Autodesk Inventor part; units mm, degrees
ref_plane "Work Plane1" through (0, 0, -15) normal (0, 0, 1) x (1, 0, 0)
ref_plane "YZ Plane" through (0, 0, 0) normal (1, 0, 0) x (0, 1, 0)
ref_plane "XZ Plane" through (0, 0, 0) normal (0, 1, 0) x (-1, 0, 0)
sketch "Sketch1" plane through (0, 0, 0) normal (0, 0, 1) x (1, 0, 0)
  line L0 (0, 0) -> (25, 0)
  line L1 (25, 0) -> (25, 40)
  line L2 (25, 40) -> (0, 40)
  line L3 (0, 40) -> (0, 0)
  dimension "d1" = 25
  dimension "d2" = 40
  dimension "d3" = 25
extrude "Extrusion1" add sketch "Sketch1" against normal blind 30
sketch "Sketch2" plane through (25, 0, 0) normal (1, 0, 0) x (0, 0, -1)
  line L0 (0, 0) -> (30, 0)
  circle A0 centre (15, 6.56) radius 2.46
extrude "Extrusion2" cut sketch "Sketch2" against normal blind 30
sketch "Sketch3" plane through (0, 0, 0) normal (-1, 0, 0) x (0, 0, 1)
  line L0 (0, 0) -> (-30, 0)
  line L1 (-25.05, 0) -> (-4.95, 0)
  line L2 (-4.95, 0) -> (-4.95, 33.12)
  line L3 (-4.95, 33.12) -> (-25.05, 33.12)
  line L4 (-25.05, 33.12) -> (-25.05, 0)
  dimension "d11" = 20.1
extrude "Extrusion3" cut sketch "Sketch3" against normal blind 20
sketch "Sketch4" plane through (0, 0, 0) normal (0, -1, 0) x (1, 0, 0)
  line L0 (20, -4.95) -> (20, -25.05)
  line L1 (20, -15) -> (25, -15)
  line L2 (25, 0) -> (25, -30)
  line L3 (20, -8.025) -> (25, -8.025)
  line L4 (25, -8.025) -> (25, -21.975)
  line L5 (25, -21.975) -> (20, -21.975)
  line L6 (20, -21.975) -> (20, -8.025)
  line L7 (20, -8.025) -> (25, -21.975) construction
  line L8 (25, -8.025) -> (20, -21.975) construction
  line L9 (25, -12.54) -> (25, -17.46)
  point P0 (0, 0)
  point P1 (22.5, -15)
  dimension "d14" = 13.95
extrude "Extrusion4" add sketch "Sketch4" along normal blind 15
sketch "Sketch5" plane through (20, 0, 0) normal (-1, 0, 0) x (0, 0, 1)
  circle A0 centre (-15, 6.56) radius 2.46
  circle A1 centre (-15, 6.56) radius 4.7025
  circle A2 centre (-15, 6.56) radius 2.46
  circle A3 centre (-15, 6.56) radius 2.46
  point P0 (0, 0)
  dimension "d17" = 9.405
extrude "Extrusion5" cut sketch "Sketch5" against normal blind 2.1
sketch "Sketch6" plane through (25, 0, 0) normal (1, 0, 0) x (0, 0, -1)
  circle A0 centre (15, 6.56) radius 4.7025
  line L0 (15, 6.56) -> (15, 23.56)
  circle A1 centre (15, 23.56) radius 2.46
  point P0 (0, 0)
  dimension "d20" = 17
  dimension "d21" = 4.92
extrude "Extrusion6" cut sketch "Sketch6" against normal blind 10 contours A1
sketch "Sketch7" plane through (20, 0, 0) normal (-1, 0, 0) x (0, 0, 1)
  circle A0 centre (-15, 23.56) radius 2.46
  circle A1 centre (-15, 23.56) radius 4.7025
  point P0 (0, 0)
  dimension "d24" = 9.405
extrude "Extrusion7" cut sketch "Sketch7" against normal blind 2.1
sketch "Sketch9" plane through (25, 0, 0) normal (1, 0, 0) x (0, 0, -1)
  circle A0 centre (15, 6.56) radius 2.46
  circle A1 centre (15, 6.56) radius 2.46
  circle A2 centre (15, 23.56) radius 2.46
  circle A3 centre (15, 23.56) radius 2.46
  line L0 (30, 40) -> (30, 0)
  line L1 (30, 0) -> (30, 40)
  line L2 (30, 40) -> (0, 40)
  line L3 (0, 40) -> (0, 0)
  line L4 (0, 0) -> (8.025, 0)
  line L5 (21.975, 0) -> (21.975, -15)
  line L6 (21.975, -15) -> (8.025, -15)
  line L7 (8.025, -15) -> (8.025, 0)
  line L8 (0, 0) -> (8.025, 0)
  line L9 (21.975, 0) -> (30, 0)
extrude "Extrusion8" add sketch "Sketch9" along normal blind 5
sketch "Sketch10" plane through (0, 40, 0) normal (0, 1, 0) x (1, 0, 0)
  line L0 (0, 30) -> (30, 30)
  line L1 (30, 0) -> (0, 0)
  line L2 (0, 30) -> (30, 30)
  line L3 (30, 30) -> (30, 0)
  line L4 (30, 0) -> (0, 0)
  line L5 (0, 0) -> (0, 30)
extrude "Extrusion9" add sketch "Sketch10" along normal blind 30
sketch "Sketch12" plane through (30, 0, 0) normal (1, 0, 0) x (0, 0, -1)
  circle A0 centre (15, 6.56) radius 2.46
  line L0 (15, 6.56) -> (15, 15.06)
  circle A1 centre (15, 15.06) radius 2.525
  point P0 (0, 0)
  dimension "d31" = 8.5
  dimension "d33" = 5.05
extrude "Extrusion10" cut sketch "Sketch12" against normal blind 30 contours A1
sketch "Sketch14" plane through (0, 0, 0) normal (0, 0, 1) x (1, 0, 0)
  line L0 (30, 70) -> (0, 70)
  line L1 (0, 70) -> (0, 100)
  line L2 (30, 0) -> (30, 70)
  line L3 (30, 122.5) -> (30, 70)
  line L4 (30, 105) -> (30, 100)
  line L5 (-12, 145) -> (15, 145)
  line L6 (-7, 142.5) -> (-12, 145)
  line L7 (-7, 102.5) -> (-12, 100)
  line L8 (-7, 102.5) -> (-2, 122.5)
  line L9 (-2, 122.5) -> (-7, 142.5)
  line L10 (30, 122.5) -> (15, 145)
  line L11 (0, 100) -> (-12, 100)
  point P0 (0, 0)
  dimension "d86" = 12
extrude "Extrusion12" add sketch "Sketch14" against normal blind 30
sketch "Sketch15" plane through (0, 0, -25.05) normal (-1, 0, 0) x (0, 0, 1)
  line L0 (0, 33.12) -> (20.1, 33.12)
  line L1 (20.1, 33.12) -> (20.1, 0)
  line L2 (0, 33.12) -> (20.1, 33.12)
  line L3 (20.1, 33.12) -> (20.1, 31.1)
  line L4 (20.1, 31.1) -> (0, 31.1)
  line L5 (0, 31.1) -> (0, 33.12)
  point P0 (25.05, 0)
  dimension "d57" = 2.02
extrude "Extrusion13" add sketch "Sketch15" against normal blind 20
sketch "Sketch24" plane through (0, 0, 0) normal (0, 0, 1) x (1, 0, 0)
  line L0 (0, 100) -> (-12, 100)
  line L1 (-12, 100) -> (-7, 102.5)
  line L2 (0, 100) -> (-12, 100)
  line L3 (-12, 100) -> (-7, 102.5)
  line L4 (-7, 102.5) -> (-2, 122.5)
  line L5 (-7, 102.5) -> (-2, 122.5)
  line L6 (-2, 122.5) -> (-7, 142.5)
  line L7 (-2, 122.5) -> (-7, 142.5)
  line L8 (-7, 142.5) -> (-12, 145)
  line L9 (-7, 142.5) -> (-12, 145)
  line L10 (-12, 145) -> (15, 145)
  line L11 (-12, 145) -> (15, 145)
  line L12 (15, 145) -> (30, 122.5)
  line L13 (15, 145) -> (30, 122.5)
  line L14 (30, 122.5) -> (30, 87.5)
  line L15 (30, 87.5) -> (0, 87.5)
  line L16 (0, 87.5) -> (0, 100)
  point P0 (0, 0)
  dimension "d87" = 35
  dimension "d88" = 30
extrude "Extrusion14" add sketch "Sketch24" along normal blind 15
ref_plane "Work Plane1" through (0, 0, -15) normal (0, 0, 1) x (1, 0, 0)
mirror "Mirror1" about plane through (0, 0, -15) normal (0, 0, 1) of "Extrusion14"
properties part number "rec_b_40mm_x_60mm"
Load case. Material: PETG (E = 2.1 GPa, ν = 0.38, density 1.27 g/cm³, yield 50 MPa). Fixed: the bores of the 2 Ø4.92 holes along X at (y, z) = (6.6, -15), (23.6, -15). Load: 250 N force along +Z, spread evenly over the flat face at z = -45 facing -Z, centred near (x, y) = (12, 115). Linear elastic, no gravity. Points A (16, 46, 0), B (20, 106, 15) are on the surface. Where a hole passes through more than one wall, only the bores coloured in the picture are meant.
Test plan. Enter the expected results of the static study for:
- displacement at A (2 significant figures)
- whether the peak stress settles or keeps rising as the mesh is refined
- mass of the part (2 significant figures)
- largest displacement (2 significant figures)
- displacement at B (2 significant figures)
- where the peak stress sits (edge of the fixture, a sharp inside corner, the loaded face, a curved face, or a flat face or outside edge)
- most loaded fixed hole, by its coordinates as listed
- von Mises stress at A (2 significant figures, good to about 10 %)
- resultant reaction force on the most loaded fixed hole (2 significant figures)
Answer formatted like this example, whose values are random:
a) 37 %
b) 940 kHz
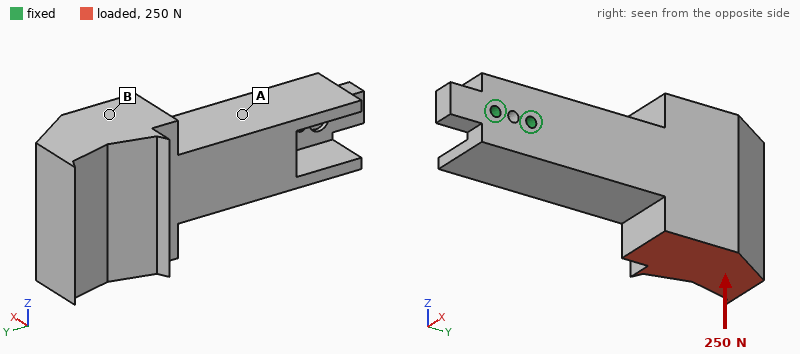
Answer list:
a) 0.35 mm
b) keeps rising
c) 220 g
d) 2.1 mm
e) 1.4 mm
f) edge of the fixture
g) (23.6, -15)
h) 4.2 MPa
i) 1.2 kN
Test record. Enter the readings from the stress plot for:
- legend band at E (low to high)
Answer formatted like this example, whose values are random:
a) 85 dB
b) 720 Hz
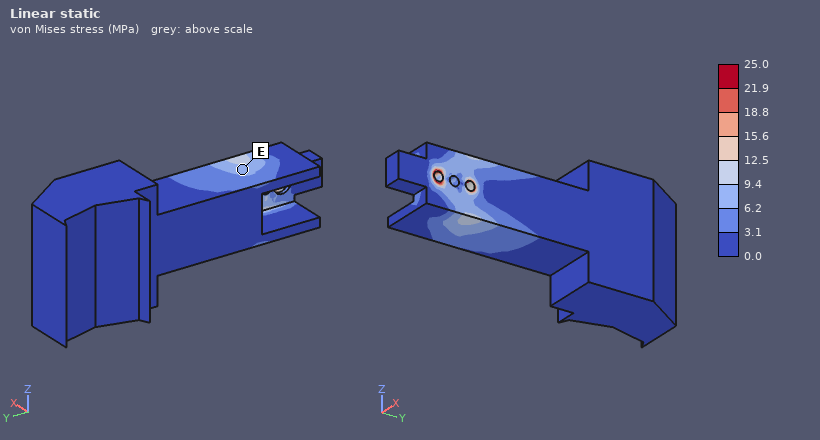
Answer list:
a) 6.2 to 9.4 MPa
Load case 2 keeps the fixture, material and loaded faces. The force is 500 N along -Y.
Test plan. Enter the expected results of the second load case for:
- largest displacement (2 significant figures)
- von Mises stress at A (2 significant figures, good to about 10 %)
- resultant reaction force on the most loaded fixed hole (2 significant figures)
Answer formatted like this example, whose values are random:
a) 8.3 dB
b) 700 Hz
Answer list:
a) 1.8 mm
b) 3.0 MPa
c) 770 N
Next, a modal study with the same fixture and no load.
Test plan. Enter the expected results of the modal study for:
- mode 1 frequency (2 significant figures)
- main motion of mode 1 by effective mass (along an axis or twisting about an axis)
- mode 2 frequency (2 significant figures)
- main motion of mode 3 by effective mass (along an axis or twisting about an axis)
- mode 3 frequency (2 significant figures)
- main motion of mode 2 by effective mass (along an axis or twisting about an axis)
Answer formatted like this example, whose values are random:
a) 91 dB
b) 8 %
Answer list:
a) 150 Hz
b) along X
c) 170 Hz
d) twisting about Y
e) 420 Hz
f) along Z
